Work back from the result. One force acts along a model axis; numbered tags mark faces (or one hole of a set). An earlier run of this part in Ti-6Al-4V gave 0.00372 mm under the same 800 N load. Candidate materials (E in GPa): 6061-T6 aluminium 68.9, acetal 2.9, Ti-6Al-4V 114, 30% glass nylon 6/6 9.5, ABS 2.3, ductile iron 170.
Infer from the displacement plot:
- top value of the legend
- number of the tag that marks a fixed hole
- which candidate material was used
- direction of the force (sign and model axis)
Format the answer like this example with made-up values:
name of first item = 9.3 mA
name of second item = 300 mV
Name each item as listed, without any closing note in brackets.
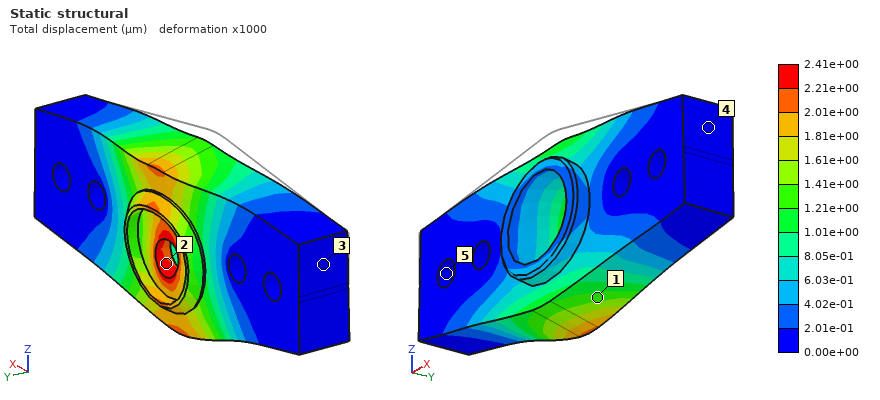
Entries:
top value of the legend = 2.41e+00 µm
number of the tag that marks a fixed hole = 5
which candidate material was used = ductile iron
direction of the force = -Z
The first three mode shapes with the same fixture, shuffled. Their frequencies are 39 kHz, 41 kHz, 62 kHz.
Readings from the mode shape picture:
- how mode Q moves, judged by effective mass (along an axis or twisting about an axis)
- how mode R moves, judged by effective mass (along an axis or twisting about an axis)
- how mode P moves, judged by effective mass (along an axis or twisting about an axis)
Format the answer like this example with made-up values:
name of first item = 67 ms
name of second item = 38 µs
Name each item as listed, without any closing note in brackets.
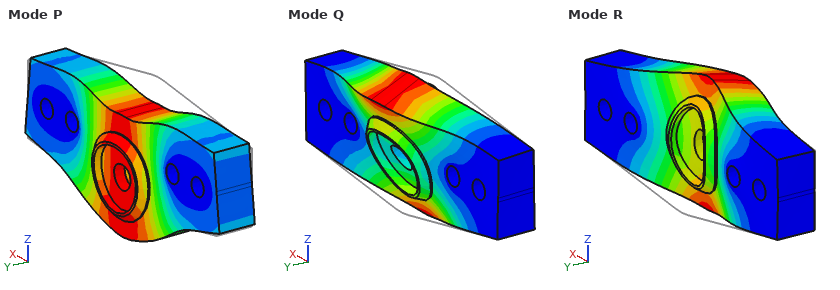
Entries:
how mode Q moves, judged by effective mass = twisting about X
how mode R moves, judged by effective mass = along Y
how mode P moves, judged by effective mass = along Z
